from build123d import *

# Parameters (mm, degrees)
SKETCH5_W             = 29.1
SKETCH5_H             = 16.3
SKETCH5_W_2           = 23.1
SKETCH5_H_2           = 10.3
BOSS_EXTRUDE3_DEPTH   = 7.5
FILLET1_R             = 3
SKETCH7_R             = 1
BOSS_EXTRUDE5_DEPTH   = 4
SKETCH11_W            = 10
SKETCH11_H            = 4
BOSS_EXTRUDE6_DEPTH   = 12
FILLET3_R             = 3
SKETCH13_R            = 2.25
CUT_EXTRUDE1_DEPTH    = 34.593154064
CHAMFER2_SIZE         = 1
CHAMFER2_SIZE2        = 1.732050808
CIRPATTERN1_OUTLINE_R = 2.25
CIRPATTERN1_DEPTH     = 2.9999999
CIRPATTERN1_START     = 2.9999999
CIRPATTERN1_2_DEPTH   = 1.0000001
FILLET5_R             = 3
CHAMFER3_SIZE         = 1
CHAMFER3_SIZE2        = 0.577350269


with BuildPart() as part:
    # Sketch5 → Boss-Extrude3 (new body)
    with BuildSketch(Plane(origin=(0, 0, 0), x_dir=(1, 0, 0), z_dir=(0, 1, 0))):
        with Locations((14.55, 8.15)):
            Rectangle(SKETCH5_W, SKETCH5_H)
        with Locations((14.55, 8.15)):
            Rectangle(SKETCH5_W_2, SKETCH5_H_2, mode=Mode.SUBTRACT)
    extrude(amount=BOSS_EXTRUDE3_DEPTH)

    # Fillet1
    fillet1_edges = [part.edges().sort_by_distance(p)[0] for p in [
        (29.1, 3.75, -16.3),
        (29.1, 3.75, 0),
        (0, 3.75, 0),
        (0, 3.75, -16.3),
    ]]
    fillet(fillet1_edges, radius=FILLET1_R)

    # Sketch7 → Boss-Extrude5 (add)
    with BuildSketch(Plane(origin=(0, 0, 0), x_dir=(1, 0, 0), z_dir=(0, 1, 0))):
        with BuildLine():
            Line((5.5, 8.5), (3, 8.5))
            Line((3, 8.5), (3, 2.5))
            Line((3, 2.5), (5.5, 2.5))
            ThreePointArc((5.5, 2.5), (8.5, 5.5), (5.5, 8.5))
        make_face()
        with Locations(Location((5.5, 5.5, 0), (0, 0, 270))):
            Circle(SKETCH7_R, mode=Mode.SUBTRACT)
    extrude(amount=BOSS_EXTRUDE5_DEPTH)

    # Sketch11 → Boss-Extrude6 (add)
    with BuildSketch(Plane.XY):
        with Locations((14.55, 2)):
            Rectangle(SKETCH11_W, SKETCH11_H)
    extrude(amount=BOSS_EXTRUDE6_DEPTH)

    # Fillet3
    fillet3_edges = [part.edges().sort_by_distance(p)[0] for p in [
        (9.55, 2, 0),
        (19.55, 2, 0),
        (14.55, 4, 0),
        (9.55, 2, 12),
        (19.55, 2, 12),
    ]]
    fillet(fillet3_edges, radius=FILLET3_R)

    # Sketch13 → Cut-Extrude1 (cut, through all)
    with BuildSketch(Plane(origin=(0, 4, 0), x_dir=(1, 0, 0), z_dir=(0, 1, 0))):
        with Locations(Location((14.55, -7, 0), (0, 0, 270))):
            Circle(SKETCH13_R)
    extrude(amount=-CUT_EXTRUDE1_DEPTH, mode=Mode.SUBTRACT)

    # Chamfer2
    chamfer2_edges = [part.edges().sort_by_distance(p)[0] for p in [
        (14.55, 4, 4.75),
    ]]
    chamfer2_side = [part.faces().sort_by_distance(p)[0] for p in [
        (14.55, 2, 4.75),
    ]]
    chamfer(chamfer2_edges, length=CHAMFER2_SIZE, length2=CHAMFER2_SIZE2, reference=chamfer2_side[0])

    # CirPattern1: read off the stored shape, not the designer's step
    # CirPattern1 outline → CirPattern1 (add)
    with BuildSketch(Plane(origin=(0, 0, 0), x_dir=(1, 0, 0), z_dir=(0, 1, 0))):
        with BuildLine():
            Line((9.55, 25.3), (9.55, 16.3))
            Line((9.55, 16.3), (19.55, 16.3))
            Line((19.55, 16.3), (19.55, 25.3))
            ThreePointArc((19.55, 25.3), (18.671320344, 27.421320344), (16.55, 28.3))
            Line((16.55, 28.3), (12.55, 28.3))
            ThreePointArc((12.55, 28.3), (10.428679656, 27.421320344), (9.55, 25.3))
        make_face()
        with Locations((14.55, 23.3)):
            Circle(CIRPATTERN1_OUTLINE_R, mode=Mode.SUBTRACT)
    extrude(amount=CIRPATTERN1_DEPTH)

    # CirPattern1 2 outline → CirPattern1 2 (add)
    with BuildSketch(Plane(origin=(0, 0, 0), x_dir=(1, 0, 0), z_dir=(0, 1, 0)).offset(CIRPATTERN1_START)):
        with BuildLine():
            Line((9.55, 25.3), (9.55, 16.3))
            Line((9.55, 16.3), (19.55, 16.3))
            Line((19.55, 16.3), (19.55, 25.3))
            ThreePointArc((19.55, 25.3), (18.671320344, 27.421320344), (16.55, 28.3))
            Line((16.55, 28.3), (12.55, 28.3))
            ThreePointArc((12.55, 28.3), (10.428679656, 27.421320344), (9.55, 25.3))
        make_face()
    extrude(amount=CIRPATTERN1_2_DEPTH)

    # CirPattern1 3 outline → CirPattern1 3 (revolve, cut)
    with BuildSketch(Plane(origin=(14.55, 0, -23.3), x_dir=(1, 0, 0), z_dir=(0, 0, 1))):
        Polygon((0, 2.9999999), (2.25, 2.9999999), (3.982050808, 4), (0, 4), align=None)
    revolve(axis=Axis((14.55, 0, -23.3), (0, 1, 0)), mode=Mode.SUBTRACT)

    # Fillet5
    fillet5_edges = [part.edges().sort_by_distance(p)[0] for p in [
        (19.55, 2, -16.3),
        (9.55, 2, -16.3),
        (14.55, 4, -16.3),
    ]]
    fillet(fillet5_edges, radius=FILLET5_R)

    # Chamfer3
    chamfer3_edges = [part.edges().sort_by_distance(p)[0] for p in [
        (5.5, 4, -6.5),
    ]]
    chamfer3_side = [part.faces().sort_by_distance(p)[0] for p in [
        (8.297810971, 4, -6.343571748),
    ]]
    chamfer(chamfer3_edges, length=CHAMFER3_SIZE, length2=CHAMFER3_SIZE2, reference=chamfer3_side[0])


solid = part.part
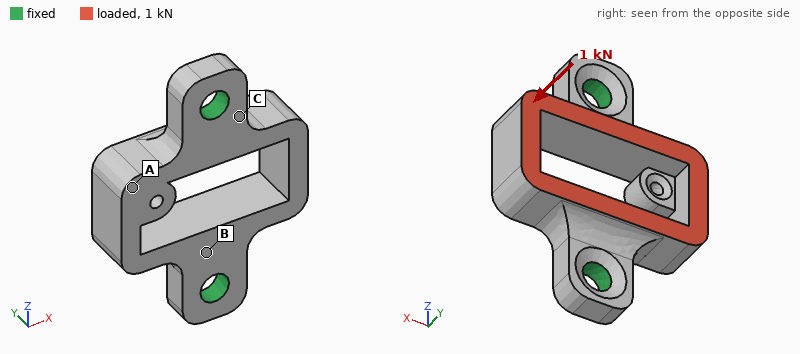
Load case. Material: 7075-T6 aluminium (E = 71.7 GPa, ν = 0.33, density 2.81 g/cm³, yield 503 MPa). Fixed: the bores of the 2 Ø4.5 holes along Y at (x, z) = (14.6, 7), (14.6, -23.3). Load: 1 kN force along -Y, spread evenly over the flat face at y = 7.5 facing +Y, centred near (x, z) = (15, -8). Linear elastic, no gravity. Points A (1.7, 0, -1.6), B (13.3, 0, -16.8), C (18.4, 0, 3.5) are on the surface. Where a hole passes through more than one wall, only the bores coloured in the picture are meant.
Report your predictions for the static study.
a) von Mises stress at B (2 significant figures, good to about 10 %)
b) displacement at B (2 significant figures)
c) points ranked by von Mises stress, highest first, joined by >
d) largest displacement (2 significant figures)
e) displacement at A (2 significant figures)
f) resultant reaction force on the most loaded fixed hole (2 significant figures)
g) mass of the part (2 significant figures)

28 MPa
12 µm
C > B > A
34 µm
28 µm
510 N
7.5 g
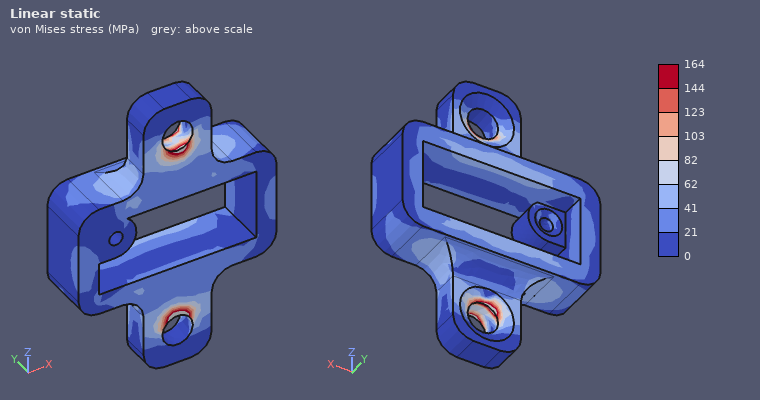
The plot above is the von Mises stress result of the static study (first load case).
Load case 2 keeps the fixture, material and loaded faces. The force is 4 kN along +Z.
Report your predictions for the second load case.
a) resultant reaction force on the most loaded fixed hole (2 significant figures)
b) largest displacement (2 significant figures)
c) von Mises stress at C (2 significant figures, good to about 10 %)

2.2 kN
61 µm
58 MPa
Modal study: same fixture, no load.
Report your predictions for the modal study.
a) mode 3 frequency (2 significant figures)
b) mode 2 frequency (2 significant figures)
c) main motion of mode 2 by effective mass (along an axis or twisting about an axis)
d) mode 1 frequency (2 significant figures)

20 kHz
14 kHz
along Y
8600 Hz
